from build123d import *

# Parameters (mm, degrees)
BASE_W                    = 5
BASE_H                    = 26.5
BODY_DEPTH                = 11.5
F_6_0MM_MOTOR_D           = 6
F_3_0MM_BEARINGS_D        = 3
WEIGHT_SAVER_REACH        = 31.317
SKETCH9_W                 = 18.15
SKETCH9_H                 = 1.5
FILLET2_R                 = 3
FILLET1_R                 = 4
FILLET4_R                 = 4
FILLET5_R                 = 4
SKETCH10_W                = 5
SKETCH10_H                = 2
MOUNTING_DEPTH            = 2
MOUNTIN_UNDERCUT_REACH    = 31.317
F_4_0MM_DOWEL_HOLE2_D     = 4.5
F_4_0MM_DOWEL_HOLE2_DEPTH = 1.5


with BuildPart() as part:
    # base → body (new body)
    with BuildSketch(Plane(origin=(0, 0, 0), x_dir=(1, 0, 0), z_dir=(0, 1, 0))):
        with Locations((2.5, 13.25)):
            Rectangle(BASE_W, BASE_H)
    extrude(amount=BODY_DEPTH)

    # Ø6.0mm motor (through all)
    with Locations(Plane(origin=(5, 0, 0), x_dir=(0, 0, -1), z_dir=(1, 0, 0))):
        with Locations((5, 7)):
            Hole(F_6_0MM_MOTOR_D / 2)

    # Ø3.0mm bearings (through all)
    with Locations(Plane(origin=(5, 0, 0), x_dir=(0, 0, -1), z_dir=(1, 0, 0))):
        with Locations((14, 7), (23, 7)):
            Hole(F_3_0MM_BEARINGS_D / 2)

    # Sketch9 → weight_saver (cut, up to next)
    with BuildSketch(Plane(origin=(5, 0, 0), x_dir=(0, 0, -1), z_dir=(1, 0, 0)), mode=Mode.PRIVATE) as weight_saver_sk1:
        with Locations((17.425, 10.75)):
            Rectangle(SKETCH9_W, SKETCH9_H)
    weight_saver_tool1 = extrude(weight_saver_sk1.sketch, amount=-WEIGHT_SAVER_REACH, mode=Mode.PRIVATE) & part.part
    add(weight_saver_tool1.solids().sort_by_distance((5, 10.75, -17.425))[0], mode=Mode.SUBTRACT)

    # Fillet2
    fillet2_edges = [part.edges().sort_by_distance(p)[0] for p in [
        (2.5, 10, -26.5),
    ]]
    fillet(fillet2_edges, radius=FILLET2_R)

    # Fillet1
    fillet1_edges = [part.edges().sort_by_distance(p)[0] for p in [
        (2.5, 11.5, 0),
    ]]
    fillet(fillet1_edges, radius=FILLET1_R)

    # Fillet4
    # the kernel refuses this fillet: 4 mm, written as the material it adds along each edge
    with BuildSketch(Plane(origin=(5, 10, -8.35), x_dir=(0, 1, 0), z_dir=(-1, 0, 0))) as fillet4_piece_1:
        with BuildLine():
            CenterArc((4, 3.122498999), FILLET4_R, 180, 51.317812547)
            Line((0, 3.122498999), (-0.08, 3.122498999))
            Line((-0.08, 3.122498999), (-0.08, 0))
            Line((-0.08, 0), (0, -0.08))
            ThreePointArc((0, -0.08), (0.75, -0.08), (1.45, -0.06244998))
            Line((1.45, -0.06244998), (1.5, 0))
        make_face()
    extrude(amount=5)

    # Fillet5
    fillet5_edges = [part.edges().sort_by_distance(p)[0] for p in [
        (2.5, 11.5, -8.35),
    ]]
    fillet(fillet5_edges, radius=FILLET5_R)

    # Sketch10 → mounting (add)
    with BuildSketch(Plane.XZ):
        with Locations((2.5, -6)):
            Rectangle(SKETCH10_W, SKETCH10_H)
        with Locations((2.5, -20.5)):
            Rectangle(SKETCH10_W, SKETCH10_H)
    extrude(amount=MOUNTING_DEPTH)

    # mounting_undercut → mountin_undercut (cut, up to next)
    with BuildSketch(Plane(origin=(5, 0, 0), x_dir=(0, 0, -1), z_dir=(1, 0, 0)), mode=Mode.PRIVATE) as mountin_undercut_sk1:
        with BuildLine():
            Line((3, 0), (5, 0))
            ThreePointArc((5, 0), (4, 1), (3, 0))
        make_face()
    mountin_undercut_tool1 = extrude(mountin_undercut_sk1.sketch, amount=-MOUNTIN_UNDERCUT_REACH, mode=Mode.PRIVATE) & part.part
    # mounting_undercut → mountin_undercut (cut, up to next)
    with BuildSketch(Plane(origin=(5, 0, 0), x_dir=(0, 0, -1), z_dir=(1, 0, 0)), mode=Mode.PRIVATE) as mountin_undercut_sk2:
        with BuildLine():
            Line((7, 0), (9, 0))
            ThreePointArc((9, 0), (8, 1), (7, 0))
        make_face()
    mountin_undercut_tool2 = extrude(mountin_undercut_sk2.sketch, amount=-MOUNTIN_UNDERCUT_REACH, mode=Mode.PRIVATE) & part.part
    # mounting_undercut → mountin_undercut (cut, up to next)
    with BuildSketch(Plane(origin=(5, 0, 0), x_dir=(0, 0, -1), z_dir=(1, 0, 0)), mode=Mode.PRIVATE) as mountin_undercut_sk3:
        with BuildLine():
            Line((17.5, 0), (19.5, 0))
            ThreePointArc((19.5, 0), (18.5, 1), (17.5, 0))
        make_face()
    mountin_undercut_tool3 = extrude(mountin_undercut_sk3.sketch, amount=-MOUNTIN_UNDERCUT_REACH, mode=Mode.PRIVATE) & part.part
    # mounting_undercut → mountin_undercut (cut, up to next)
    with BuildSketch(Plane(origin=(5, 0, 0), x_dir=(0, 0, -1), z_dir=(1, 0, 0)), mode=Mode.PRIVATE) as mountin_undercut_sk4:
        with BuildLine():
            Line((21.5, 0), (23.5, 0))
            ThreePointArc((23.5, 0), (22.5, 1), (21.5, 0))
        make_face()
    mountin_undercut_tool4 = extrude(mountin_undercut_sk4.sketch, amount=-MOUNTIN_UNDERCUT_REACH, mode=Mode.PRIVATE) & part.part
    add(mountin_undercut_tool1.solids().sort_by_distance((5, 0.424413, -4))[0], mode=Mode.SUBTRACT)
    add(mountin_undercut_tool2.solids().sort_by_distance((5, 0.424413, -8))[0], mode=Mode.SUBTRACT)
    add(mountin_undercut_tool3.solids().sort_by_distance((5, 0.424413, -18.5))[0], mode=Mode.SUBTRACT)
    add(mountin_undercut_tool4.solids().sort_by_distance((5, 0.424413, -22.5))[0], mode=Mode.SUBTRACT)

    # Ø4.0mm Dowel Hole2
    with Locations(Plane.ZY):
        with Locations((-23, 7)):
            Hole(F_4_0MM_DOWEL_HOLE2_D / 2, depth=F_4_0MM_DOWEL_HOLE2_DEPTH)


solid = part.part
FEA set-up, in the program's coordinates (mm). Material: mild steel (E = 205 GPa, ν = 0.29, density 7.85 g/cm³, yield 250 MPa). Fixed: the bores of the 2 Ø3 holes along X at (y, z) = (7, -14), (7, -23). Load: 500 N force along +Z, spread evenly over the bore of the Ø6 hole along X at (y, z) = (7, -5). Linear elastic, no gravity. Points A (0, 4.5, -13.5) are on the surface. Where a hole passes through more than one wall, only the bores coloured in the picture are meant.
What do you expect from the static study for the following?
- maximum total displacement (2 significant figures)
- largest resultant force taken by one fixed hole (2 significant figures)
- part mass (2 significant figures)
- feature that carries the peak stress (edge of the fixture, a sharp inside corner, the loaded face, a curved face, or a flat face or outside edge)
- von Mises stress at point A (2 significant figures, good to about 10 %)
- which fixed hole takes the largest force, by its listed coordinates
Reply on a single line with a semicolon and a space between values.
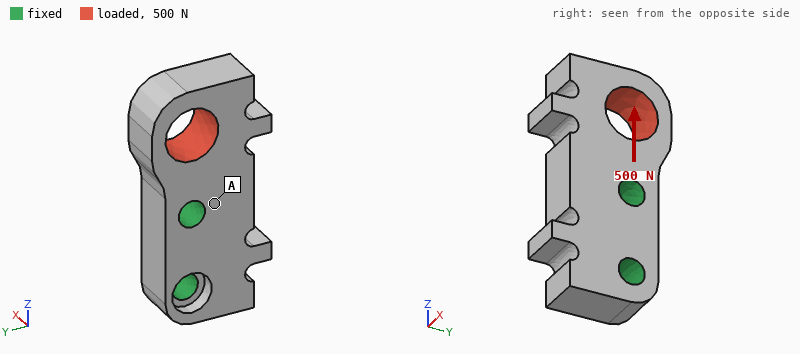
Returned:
2.3 µm; 470 N; 9.0 g; the loaded face; 4.7 MPa; (7, -14)
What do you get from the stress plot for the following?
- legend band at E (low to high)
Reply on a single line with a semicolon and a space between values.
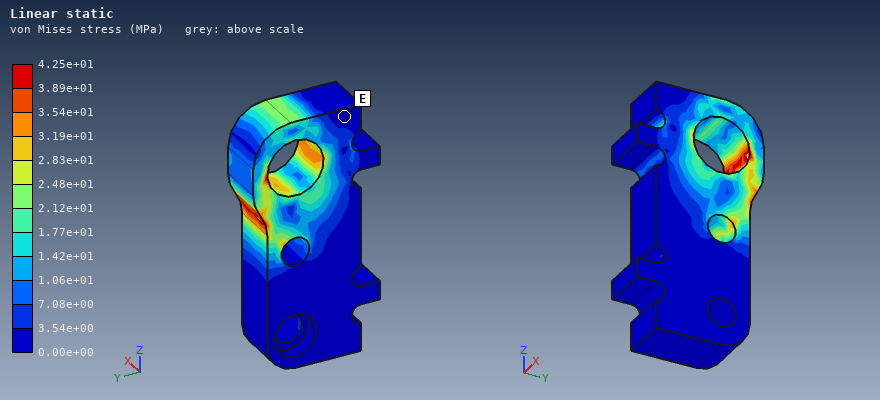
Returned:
0.00e+00 to 3.54e+00 MPa
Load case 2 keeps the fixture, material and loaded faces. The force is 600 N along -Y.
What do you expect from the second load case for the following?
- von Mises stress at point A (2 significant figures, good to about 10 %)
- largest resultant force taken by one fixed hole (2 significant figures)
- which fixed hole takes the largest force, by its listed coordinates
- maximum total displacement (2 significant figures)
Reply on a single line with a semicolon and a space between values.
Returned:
30 MPa; 920 N; (7, -14); 12 µm
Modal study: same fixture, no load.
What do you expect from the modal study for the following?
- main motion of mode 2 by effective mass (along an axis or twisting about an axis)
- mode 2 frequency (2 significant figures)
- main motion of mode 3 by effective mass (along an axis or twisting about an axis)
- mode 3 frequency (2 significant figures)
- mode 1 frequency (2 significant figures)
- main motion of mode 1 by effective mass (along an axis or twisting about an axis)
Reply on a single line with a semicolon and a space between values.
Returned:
along Y; 23 kHz; twisting about Z; 35 kHz; 19 kHz; along X
